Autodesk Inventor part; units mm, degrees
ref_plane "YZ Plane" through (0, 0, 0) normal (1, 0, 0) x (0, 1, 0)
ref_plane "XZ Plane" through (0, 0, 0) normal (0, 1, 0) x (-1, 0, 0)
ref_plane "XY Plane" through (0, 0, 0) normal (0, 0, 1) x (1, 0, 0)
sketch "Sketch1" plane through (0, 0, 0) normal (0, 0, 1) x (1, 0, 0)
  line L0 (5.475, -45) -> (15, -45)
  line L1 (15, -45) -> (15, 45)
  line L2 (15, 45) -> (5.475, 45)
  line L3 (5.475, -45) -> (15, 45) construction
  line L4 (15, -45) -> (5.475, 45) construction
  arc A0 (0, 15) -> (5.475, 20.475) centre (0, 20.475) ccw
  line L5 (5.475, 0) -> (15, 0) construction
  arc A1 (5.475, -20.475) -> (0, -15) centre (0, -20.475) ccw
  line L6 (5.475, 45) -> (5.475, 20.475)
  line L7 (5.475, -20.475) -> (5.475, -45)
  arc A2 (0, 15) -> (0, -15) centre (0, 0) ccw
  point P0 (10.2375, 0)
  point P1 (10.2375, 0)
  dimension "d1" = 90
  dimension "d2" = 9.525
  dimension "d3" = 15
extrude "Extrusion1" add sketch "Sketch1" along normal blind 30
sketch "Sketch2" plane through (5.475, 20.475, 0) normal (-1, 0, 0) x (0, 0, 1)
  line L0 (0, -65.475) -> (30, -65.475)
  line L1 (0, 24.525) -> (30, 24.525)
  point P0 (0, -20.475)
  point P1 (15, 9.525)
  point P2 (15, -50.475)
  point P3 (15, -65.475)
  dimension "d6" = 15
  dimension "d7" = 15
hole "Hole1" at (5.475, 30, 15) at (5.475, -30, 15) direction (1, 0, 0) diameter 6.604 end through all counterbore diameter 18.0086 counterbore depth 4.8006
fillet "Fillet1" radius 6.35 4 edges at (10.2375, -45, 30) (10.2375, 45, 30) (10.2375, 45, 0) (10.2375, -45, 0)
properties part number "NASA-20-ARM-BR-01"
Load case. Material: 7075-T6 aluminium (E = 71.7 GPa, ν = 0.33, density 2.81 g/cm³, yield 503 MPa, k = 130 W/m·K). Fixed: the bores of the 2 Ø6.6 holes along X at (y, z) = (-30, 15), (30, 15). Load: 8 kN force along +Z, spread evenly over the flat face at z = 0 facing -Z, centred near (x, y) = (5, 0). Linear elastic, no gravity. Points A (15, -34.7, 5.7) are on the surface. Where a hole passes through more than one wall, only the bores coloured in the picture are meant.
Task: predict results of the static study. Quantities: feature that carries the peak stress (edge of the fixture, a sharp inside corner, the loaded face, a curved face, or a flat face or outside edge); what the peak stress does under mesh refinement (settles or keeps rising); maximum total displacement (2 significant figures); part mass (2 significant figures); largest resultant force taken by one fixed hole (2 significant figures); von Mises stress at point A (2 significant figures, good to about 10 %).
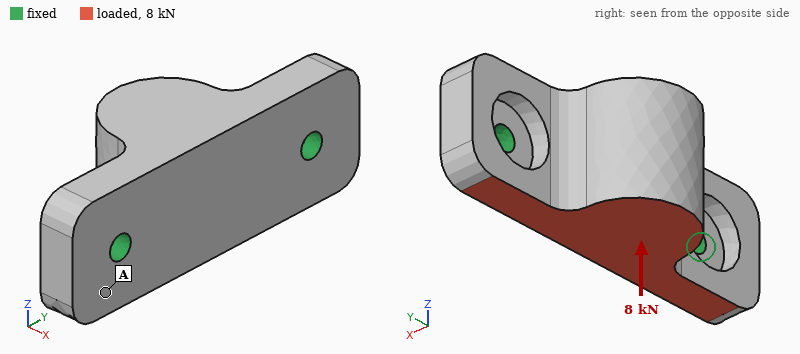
edge of the fixture
keeps rising
0.19 mm
110 g
4.0 kN
56 MPa
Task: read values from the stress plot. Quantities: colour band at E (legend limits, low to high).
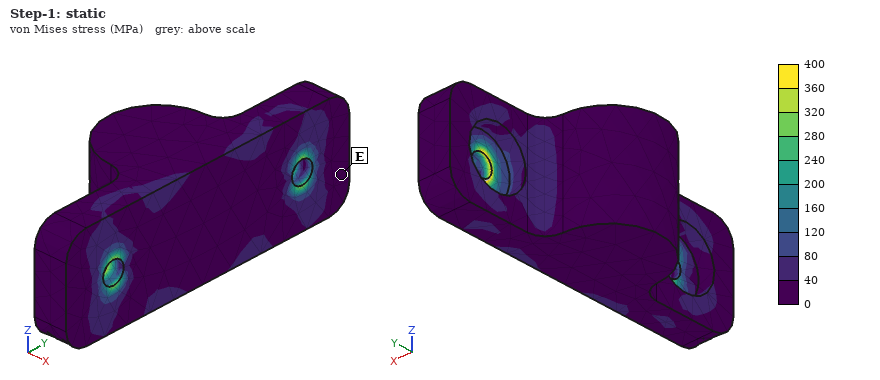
0 to 40 MPa
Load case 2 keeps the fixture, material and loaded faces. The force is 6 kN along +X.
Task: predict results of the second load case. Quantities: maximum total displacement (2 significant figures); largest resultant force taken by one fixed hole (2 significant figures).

0.23 mm
3.5 kN
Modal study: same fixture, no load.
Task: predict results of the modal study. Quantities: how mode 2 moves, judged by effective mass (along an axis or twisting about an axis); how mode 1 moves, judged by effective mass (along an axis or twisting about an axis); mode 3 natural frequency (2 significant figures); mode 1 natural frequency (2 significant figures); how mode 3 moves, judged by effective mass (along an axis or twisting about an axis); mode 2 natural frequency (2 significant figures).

along X
along Z
13 kHz
3700 Hz
along Y
7900 Hz
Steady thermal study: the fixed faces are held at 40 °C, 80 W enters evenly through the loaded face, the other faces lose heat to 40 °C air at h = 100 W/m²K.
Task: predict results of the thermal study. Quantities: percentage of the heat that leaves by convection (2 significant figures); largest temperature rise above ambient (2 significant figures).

15 %
28 K
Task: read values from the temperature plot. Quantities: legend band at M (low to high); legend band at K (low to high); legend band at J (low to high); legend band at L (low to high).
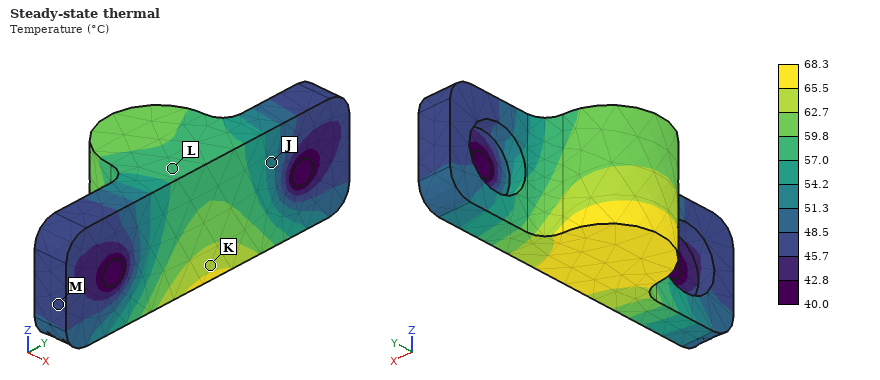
45.7 to 48.5 °C
62.7 to 65.5 °C
51.3 to 54.2 °C
57.0 to 59.8 °C
